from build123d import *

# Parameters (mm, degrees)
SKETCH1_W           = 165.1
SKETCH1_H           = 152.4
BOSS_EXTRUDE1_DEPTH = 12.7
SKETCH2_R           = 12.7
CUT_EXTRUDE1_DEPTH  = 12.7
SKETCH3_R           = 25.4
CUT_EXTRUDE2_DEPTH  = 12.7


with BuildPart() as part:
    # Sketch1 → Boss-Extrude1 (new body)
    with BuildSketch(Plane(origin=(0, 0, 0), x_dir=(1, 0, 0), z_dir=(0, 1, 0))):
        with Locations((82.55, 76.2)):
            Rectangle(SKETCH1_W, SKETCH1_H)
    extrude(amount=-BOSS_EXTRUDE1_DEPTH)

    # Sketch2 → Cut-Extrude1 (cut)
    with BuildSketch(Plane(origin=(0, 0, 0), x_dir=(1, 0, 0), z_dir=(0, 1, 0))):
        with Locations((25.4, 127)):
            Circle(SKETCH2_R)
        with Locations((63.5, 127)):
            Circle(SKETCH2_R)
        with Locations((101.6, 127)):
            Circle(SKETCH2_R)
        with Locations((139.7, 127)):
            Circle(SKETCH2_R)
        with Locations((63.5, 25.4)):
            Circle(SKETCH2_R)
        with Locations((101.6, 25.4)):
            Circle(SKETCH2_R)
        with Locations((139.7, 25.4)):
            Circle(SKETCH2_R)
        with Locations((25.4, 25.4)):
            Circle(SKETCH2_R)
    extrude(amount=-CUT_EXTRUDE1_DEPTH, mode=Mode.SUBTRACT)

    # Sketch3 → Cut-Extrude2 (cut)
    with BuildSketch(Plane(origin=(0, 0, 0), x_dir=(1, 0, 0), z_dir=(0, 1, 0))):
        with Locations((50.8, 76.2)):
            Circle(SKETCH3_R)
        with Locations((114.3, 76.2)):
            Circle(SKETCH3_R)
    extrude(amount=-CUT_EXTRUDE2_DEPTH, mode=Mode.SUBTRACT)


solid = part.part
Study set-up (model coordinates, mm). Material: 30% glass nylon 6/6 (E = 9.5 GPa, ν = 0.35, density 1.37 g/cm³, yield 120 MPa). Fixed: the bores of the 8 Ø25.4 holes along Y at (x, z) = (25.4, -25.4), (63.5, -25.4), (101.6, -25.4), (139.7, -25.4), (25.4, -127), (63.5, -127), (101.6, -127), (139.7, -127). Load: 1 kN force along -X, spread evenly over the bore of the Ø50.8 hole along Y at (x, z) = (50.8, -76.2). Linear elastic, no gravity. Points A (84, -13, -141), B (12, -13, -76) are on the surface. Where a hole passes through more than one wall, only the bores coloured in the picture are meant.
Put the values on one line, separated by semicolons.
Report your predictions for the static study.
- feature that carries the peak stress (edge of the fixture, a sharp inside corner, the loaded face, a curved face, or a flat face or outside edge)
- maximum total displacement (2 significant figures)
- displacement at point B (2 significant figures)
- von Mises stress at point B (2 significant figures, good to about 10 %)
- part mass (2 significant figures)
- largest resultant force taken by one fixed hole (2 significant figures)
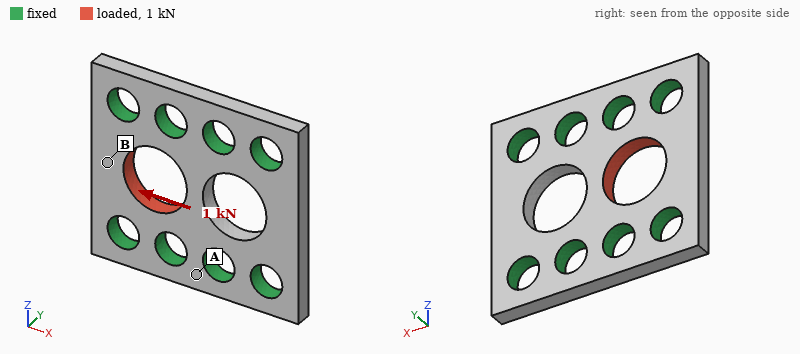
edge of the fixture; 5.1 µm; 4.6 µm; 0.41 MPa; 300 g; 200 N
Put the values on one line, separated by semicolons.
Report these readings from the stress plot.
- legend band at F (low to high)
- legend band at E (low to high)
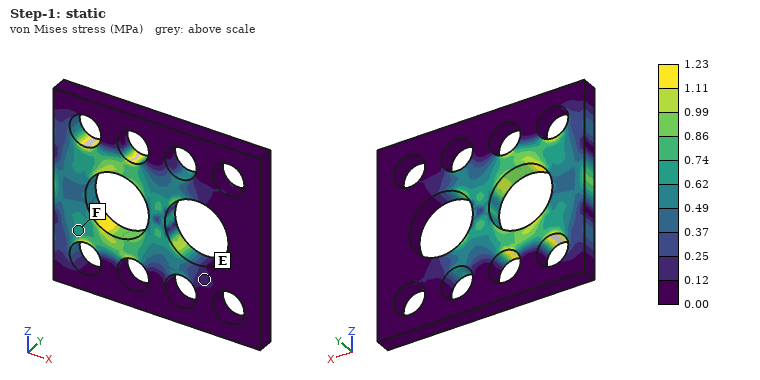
0.62 to 0.74 MPa; 0.12 to 0.25 MPa
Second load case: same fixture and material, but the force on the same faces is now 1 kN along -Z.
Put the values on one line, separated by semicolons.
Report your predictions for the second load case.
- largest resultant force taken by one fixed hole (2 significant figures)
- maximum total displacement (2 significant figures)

230 N; 2.0 µm
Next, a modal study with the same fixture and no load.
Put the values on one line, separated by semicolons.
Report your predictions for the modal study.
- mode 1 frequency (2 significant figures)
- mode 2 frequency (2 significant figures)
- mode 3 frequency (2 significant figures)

4500 Hz; 4500 Hz; 6000 Hz
